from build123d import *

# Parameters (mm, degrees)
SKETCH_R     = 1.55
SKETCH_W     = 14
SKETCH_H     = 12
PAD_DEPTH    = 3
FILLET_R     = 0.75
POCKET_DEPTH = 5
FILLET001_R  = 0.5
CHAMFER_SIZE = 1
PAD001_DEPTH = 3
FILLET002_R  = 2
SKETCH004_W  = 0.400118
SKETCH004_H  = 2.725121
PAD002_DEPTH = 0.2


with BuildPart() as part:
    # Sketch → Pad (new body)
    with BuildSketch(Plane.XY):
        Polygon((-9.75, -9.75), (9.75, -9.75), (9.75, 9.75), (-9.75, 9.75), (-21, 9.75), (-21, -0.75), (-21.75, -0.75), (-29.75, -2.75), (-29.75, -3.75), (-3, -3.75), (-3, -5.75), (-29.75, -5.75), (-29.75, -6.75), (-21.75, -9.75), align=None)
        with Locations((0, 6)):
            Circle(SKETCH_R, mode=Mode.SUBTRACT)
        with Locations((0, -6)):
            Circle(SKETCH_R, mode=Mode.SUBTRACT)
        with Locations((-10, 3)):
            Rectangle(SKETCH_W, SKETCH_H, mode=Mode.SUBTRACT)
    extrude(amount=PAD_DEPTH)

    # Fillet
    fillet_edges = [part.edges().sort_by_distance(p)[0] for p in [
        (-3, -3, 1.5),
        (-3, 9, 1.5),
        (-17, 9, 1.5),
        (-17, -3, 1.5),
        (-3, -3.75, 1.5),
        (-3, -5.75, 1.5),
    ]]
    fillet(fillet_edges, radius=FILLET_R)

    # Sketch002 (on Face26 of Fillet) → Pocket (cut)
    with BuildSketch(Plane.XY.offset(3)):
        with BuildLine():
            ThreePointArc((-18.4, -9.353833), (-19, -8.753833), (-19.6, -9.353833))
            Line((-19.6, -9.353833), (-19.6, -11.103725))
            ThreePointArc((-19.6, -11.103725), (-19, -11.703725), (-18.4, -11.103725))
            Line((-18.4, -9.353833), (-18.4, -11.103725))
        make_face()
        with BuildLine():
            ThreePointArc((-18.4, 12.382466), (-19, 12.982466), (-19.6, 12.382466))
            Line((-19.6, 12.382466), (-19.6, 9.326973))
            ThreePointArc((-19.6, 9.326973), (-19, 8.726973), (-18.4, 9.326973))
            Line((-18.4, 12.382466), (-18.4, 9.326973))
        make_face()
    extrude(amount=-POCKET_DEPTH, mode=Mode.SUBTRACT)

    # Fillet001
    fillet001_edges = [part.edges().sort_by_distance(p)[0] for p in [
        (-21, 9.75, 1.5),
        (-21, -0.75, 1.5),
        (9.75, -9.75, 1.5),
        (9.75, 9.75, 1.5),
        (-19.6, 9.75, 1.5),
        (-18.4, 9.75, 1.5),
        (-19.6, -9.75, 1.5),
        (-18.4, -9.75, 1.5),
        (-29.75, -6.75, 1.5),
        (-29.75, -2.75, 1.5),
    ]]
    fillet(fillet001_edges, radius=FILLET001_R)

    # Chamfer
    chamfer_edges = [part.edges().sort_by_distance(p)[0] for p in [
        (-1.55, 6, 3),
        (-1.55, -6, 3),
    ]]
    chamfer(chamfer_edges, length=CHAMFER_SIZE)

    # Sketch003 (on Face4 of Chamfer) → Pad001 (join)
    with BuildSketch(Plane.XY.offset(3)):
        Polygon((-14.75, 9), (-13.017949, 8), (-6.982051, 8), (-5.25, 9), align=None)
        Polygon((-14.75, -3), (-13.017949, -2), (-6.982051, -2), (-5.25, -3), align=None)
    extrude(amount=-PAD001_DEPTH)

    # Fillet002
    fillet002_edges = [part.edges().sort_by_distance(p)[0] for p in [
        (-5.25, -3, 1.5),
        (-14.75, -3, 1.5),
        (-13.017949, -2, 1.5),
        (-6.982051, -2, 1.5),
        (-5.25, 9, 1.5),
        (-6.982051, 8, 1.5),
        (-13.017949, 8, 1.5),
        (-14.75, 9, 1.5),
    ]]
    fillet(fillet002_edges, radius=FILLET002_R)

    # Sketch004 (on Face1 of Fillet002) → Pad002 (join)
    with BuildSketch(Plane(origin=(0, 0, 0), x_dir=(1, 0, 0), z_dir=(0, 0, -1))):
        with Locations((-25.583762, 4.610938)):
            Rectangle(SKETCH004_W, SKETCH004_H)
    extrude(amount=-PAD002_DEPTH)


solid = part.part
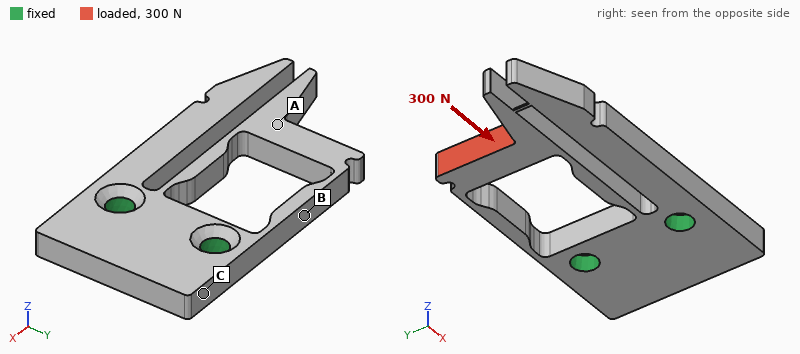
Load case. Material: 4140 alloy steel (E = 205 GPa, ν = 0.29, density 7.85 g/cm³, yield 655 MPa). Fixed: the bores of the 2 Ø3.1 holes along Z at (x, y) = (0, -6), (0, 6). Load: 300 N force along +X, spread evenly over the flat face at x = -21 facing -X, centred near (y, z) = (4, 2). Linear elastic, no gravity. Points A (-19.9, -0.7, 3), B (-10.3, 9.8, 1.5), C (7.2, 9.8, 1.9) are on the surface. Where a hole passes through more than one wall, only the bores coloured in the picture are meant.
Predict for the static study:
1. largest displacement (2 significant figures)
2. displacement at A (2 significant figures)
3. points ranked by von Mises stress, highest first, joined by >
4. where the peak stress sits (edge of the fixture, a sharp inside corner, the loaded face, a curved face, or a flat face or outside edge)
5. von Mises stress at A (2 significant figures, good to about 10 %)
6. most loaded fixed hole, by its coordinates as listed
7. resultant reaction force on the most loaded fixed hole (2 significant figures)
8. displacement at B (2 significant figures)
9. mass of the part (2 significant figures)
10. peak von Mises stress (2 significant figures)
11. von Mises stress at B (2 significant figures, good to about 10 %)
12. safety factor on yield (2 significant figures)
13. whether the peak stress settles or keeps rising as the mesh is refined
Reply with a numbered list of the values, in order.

1. 9.1 µm
2. 6.5 µm
3. B > A > C
4. a curved face
5. 31 MPa
6. (0, 6)
7. 220 N
8. 4.5 µm
9. 10 g
10. 190 MPa
11. 81 MPa
12. 3.5
13. settles
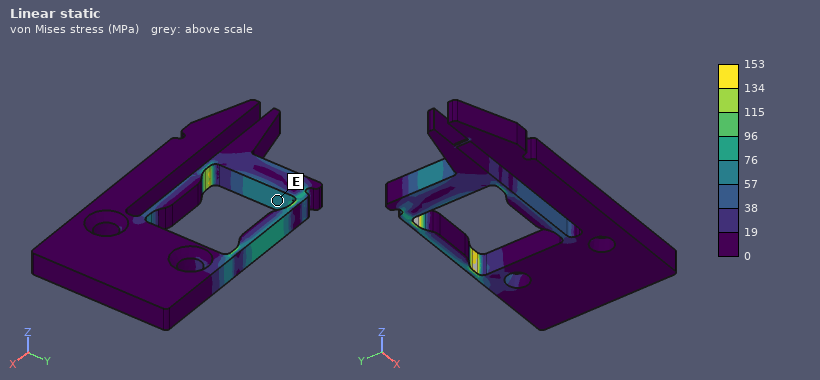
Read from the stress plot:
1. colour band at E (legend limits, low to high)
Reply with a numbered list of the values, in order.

1. 57 to 76 MPa
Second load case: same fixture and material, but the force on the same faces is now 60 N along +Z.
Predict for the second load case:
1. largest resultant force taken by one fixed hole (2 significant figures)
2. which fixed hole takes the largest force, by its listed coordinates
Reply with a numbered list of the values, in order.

1. 34 N
2. (0, 6)
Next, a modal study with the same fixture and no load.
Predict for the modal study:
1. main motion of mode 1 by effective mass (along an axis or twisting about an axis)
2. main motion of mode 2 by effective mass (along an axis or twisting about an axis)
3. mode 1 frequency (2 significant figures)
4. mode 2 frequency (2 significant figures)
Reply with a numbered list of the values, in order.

1. along Z
2. along Y
3. 2600 Hz
4. 2800 Hz
